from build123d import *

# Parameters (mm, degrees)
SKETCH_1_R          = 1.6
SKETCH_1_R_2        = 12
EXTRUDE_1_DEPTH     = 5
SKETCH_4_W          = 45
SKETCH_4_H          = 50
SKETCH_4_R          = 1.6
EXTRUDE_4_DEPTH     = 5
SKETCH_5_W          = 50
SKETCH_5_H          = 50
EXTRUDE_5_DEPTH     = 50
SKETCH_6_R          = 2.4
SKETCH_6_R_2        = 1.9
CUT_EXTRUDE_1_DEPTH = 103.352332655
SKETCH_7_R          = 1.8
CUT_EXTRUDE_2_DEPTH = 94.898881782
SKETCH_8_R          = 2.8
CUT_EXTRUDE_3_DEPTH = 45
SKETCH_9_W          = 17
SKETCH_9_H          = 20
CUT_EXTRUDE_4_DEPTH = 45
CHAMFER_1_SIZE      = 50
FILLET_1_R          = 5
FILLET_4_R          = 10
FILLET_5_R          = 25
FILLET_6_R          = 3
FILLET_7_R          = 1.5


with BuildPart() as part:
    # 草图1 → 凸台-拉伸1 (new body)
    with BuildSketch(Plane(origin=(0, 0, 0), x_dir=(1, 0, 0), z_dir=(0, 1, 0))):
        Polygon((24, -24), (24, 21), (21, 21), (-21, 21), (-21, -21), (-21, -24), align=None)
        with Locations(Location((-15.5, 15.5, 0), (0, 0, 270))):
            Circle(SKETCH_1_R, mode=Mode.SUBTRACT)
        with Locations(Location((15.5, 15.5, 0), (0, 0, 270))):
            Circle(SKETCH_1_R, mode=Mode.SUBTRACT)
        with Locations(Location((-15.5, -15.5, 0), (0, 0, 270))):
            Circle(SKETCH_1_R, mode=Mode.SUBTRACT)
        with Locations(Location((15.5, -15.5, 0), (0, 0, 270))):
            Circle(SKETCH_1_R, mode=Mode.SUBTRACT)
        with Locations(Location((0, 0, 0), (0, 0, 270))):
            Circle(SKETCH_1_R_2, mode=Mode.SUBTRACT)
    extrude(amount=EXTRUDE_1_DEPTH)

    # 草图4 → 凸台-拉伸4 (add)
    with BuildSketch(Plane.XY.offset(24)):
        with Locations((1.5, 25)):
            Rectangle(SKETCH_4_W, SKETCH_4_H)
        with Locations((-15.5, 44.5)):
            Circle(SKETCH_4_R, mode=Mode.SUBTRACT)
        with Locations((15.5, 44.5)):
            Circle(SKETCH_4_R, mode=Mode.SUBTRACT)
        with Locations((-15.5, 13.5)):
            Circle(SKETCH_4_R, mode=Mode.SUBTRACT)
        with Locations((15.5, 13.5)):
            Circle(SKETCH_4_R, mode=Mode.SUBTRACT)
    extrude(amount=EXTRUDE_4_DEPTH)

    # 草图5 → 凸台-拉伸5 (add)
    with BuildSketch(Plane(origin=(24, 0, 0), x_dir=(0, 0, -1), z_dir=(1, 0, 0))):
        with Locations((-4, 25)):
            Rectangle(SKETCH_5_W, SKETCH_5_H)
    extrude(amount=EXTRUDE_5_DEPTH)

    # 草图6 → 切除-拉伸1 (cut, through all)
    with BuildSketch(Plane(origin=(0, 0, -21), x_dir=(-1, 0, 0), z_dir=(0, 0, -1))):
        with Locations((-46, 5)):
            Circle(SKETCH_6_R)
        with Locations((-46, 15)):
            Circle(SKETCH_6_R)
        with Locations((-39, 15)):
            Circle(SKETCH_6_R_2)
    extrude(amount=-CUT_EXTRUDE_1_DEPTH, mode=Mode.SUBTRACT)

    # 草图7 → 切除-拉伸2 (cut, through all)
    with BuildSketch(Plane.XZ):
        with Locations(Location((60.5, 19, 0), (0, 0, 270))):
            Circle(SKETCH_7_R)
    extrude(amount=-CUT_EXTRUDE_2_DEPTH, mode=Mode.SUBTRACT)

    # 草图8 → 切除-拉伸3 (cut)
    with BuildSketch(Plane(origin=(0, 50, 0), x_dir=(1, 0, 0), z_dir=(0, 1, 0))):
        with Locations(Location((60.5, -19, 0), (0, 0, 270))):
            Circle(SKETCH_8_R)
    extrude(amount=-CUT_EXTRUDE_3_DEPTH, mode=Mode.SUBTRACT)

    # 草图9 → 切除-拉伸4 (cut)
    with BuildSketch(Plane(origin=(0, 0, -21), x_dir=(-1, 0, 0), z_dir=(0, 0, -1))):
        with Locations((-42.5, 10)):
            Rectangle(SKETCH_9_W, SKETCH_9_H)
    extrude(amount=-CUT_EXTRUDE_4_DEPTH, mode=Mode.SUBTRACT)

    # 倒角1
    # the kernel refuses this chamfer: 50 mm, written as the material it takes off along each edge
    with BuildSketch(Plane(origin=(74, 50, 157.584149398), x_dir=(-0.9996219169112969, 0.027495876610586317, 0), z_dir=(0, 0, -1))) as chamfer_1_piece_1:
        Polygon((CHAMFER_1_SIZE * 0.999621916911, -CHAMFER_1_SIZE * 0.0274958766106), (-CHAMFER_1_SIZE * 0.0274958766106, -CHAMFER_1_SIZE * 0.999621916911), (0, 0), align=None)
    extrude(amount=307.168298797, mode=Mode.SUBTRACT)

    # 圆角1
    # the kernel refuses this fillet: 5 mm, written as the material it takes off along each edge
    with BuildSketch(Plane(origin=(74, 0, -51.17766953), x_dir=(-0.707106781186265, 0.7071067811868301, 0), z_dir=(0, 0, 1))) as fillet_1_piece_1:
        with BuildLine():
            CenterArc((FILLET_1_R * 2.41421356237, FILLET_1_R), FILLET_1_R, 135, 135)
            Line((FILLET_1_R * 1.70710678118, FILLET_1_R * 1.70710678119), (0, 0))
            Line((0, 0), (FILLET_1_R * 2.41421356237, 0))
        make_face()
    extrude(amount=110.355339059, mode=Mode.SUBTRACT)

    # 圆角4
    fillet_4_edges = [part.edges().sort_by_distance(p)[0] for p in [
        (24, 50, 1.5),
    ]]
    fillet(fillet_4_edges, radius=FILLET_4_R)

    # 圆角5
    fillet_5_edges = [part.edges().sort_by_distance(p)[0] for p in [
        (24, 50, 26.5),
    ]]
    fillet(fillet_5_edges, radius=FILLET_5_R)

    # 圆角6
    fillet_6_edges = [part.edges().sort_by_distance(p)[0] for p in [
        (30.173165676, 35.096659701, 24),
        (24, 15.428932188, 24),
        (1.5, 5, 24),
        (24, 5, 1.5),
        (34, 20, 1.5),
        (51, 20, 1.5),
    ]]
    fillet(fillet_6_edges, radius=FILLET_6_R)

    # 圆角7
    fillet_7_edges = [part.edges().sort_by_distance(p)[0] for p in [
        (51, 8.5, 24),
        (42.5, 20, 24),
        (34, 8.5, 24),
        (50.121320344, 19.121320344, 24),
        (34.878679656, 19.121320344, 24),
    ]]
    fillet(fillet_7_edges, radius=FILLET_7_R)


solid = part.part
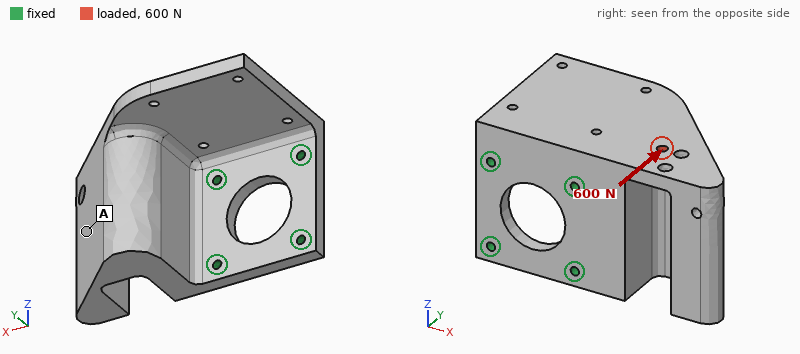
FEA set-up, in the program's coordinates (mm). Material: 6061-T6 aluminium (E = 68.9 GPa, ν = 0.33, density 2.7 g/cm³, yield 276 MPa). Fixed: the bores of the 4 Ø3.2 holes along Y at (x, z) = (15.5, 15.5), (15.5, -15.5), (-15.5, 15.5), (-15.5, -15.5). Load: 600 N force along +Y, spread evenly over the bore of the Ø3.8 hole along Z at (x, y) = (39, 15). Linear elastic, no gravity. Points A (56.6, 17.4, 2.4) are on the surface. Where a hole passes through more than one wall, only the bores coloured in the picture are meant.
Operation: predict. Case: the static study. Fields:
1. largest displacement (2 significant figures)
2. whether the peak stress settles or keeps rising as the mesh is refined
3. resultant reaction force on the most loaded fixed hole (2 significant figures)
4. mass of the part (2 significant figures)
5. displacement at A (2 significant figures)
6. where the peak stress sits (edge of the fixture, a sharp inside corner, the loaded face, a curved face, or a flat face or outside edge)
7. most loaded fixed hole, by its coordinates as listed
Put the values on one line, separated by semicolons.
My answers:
50 µm; keeps rising; 1.2 kN; 160 g; 32 µm; edge of the fixture; (15.5, 15.5)
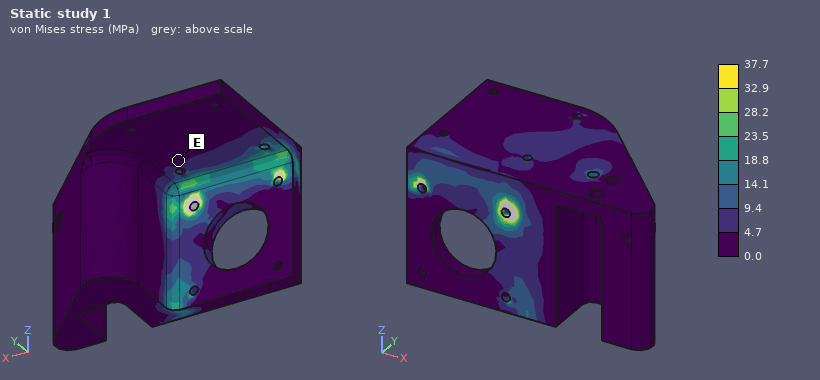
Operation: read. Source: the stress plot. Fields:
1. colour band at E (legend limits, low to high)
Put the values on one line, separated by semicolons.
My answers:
0.0 to 4.7 MPa
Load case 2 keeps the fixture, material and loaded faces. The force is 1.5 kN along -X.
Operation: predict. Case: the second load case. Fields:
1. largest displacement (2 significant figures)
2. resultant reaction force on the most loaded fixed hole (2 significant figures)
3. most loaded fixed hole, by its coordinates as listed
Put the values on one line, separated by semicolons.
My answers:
44 µm; 1.2 kN; (15.5, 15.5)
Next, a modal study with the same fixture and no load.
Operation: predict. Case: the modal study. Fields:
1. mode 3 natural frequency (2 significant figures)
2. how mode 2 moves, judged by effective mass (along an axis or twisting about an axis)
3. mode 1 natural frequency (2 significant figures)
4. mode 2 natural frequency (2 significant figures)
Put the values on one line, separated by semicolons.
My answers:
3500 Hz; along Z; 1900 Hz; 2500 Hz
